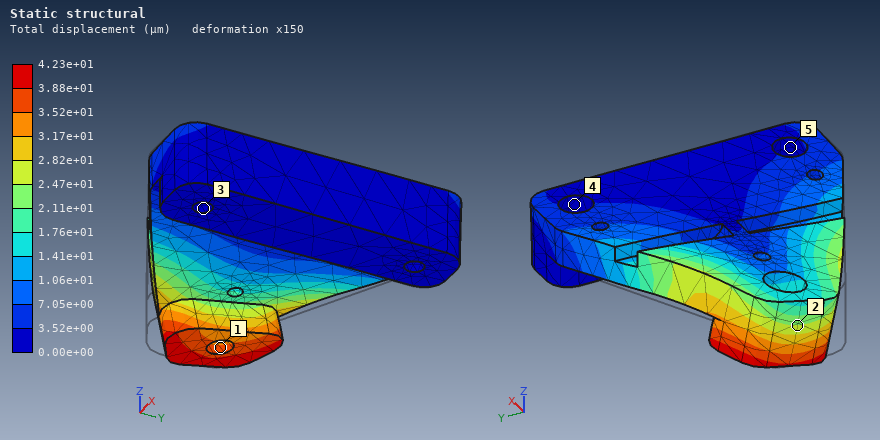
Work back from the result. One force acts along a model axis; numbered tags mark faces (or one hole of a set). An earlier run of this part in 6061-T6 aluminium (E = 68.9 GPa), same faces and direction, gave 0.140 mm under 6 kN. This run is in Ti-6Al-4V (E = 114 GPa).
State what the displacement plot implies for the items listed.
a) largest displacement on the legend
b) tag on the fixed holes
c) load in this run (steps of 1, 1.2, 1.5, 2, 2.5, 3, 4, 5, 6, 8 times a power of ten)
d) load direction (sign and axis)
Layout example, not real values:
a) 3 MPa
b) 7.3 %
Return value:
a) 4.23e+01 µm
b) 3
c) 3 kN
d) +Y
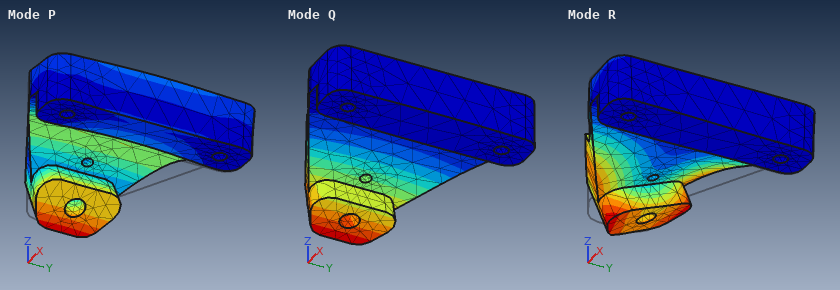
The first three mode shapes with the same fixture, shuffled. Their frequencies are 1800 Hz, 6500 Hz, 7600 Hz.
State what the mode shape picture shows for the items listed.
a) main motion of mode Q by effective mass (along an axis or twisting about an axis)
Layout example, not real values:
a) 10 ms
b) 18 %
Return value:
a) along Z
